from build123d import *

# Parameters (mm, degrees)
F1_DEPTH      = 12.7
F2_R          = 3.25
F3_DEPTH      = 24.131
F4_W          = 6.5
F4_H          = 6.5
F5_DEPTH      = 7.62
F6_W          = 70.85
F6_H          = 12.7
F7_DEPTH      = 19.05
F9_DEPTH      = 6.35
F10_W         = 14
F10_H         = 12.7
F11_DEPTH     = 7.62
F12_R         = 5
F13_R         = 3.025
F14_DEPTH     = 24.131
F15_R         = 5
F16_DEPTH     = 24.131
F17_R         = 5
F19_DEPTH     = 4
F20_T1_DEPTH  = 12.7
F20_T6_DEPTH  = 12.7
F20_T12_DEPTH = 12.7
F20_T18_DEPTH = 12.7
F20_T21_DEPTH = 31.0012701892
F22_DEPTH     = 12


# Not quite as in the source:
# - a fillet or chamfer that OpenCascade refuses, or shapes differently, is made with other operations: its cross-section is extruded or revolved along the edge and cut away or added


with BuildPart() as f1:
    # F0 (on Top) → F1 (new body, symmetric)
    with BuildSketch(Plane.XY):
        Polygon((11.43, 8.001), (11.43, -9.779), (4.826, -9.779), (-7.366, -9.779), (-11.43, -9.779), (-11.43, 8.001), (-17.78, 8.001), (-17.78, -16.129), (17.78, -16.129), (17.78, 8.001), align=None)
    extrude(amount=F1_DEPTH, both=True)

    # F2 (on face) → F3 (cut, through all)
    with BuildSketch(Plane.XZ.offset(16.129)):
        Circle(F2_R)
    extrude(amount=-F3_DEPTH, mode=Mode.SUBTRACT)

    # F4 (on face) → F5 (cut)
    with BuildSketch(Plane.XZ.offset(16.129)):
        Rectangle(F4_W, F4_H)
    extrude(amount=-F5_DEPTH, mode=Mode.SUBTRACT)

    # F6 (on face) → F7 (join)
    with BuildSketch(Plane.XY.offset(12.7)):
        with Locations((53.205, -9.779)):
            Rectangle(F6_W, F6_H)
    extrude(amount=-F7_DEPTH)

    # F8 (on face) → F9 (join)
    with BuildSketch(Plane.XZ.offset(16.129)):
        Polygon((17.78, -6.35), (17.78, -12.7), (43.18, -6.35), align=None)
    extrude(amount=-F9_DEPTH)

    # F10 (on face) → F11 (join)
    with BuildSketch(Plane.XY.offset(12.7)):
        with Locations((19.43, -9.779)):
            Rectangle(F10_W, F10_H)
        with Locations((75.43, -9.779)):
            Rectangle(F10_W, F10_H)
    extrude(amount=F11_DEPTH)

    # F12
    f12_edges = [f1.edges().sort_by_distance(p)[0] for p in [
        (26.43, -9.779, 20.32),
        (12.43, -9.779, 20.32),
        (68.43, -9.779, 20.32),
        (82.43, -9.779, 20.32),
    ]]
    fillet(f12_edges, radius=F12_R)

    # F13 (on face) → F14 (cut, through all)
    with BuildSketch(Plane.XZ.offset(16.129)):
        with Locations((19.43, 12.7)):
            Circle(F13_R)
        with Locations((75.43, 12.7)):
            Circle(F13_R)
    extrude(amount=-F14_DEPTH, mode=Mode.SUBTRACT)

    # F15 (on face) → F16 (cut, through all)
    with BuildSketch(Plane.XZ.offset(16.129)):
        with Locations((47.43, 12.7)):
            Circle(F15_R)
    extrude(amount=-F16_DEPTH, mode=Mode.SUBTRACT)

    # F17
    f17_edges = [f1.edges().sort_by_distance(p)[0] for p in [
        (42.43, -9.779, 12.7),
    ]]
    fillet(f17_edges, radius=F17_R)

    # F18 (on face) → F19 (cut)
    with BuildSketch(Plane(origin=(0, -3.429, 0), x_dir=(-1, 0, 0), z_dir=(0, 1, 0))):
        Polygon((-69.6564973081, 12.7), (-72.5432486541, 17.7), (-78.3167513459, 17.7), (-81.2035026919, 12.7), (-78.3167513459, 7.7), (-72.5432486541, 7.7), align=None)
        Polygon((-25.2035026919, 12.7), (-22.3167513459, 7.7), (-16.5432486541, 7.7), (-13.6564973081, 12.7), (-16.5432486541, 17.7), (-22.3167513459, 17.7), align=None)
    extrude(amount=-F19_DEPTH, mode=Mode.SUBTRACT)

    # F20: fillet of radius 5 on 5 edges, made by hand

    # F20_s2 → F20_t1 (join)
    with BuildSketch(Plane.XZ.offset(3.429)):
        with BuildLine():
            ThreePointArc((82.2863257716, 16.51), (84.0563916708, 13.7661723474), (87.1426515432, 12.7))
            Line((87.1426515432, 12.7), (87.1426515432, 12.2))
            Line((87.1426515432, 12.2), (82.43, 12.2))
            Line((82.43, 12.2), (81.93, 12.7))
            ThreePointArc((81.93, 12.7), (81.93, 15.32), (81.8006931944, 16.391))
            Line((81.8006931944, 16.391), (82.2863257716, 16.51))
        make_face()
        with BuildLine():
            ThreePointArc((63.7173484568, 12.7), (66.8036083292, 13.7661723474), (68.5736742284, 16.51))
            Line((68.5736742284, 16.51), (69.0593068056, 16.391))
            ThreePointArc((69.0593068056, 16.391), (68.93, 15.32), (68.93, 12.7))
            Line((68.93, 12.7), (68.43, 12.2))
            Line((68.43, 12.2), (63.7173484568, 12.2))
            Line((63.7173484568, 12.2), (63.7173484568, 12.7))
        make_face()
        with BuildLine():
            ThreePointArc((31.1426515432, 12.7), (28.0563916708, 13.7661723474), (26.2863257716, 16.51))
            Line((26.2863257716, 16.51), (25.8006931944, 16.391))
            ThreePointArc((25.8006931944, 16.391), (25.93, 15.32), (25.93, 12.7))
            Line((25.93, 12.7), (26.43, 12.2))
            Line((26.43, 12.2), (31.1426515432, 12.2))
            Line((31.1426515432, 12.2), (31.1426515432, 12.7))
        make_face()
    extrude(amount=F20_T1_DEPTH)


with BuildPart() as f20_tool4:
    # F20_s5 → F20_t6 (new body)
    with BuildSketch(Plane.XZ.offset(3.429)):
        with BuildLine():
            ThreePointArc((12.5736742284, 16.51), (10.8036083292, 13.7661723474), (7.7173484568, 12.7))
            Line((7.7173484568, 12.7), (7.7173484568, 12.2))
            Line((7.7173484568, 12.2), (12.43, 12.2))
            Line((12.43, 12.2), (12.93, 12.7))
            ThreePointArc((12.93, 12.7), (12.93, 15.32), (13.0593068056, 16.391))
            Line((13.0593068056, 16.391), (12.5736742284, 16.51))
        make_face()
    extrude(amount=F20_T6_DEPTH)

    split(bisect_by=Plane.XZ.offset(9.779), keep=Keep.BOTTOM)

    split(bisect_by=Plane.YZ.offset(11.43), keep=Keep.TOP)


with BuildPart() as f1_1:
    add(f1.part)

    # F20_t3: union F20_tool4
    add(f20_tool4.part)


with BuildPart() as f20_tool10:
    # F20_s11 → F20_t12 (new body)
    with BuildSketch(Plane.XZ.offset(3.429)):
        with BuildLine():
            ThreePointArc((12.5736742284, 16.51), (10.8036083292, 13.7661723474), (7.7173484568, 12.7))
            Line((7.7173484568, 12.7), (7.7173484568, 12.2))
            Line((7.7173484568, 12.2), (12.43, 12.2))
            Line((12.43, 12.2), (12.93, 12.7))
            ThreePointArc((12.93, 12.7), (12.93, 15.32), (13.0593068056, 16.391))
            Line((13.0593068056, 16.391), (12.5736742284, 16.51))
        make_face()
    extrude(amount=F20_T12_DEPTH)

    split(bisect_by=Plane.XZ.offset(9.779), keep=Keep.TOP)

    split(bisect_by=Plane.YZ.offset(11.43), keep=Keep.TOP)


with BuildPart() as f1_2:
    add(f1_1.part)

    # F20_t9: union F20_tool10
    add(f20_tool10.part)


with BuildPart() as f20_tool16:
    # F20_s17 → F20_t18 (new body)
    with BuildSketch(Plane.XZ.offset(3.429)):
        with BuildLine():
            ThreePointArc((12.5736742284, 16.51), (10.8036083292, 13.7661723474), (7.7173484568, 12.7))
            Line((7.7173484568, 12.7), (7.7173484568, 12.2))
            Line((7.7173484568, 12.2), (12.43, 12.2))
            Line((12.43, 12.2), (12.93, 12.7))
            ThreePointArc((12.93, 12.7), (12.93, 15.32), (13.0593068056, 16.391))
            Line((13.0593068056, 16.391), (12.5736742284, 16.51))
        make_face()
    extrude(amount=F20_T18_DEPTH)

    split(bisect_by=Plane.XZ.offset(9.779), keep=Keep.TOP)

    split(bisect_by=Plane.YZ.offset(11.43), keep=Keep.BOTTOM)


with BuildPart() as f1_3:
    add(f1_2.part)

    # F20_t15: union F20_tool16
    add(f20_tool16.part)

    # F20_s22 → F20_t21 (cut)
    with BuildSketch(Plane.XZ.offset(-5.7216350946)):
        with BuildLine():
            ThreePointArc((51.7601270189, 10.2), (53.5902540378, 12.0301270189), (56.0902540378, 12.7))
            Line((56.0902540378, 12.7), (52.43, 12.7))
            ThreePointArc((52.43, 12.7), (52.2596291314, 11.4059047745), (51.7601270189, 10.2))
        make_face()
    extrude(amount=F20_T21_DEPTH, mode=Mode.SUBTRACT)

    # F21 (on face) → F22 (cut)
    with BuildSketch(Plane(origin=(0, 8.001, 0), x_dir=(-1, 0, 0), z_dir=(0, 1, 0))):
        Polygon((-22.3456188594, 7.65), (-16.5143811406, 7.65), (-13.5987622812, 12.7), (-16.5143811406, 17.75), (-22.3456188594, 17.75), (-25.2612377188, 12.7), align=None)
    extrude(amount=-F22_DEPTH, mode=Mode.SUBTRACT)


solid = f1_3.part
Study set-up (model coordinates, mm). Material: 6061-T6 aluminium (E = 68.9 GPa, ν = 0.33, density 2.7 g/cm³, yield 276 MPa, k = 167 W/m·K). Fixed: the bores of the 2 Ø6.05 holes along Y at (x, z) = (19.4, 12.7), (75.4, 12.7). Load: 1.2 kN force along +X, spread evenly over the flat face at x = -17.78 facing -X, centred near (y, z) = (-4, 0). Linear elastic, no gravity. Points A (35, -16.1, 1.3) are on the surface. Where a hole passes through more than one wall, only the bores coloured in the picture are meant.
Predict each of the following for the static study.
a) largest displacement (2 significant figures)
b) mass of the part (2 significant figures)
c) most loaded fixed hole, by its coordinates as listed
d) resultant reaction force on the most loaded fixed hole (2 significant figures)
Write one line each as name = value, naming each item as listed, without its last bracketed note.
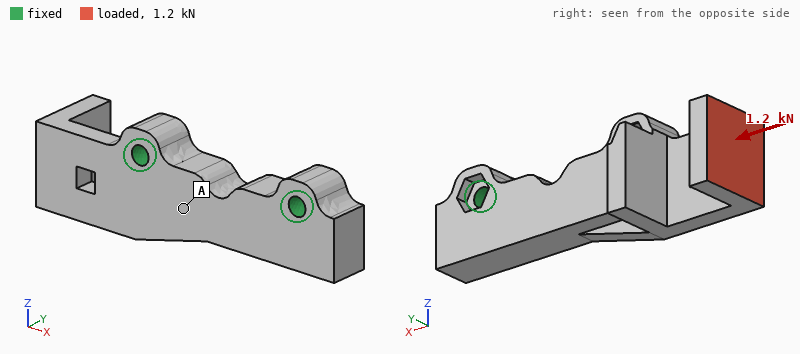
largest displacement = 0.28 mm
mass of the part = 80 g
most loaded fixed hole, by its coordinates as listed = (19.4, 12.7)
resultant reaction force on the most loaded fixed hole = 750 N
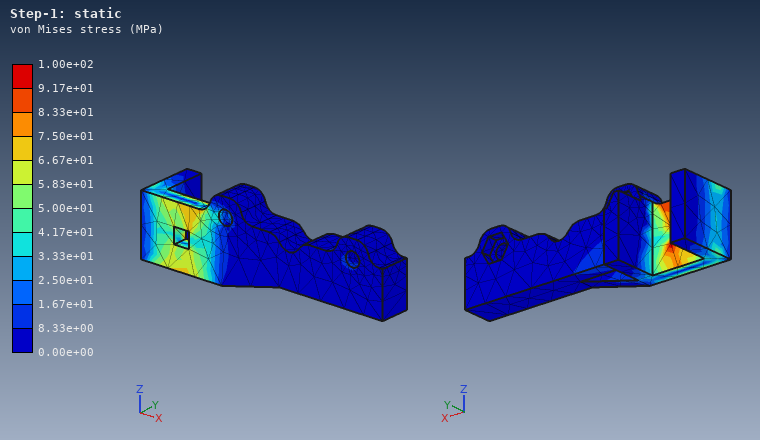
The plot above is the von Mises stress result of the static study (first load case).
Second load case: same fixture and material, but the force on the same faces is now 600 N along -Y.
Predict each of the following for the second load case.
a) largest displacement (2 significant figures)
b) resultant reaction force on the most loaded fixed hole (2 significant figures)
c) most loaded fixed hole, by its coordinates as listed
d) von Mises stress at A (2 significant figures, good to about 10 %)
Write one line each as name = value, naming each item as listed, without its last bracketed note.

largest displacement = 0.32 mm
resultant reaction force on the most loaded fixed hole = 800 N
most loaded fixed hole, by its coordinates as listed = (19.4, 12.7)
von Mises stress at A = 9.9 MPa
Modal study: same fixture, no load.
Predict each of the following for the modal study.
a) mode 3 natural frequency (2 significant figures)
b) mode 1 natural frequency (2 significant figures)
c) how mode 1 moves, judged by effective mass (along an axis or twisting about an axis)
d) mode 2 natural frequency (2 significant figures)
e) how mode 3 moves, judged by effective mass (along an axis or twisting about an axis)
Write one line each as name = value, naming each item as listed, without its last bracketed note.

mode 3 natural frequency = 7300 Hz
mode 1 natural frequency = 2400 Hz
how mode 1 moves, judged by effective mass = along Y
mode 2 natural frequency = 4100 Hz
how mode 3 moves, judged by effective mass = along Y
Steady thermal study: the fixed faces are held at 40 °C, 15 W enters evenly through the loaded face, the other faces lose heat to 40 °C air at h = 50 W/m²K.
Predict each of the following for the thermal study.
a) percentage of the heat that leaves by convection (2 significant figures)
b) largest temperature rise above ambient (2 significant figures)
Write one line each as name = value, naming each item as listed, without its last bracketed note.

percentage of the heat that leaves by convection = 16 %
largest temperature rise above ambient = 23 K
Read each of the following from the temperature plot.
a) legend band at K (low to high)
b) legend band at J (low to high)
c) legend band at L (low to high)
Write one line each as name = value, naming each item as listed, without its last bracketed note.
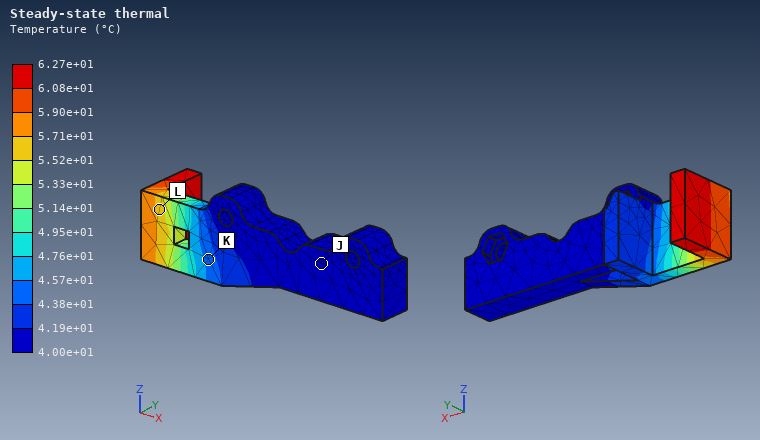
legend band at K = 4.38e+01 to 4.57e+01 °C
legend band at J = 4.00e+01 to 4.19e+01 °C
legend band at L = 5.52e+01 to 5.71e+01 °C
